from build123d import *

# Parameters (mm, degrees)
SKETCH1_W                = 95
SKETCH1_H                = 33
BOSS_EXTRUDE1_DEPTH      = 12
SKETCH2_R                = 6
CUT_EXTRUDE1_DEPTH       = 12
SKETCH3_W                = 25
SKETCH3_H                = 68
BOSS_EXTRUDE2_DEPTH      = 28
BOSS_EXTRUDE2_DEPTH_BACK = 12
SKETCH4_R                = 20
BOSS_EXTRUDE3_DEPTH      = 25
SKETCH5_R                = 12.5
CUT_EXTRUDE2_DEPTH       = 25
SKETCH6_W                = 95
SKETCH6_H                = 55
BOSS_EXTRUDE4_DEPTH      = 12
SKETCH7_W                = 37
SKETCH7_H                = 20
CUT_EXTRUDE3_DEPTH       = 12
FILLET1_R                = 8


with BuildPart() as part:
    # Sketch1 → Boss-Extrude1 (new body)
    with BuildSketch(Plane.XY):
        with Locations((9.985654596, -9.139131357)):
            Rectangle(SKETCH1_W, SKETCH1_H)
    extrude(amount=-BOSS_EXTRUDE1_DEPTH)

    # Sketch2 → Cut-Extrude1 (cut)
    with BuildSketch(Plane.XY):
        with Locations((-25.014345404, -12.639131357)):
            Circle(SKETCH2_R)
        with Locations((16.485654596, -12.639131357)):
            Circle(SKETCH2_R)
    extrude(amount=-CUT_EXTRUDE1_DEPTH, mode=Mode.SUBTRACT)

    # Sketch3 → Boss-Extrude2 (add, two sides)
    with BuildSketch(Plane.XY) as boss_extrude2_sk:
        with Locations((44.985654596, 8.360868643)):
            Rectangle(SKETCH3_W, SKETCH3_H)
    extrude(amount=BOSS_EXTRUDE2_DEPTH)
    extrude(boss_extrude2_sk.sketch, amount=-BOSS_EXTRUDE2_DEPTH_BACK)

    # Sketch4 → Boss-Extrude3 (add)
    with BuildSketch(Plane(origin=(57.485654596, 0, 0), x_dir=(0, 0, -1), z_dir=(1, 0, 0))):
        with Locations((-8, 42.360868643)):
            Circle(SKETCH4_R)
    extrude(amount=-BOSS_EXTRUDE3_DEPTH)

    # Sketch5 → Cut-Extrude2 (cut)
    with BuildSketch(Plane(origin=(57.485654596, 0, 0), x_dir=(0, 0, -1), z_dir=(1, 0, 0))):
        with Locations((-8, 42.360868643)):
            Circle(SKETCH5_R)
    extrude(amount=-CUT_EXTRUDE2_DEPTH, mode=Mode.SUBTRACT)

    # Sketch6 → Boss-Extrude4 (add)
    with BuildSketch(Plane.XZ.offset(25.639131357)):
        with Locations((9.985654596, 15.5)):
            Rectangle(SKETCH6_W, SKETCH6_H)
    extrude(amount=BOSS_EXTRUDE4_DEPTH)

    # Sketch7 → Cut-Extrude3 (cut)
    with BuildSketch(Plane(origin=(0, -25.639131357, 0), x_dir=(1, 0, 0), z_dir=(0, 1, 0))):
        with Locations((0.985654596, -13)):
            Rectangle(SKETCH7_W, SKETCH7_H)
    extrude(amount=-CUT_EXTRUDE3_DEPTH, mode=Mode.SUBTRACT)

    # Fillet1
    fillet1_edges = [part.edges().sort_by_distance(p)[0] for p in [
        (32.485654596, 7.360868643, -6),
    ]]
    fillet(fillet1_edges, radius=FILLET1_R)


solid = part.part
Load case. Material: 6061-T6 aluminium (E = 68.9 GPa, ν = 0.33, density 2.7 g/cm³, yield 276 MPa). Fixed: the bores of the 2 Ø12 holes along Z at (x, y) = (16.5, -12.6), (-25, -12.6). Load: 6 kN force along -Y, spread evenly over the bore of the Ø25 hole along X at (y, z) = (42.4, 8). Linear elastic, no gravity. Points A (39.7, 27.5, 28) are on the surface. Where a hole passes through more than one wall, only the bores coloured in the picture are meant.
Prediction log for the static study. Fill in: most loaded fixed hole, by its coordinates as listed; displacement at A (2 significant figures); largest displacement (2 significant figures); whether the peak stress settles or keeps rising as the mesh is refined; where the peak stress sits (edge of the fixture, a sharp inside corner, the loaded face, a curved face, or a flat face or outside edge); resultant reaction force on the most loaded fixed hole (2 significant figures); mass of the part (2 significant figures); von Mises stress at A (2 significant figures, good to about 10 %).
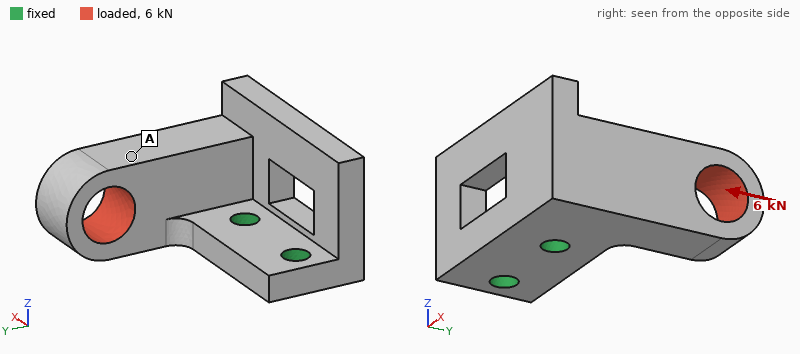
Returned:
(16.5, -12.6)
0.10 mm
0.14 mm
keeps rising
edge of the fixture
8.3 kN
410 g
11 MPa
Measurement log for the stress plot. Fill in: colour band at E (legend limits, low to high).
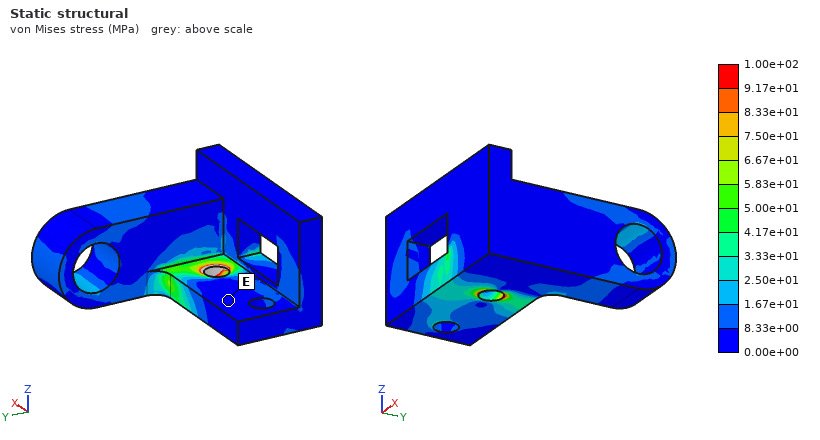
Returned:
0.00e+00 to 8.33e+00 MPa
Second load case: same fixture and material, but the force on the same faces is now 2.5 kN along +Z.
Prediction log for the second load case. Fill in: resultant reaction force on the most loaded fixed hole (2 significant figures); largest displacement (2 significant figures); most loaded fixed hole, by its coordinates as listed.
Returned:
3.1 kN
0.25 mm
(16.5, -12.6)
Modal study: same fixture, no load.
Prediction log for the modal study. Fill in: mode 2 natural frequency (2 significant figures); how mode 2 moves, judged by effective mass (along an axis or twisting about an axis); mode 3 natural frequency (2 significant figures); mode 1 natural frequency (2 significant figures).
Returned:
2400 Hz
along X
3500 Hz
1800 Hz
